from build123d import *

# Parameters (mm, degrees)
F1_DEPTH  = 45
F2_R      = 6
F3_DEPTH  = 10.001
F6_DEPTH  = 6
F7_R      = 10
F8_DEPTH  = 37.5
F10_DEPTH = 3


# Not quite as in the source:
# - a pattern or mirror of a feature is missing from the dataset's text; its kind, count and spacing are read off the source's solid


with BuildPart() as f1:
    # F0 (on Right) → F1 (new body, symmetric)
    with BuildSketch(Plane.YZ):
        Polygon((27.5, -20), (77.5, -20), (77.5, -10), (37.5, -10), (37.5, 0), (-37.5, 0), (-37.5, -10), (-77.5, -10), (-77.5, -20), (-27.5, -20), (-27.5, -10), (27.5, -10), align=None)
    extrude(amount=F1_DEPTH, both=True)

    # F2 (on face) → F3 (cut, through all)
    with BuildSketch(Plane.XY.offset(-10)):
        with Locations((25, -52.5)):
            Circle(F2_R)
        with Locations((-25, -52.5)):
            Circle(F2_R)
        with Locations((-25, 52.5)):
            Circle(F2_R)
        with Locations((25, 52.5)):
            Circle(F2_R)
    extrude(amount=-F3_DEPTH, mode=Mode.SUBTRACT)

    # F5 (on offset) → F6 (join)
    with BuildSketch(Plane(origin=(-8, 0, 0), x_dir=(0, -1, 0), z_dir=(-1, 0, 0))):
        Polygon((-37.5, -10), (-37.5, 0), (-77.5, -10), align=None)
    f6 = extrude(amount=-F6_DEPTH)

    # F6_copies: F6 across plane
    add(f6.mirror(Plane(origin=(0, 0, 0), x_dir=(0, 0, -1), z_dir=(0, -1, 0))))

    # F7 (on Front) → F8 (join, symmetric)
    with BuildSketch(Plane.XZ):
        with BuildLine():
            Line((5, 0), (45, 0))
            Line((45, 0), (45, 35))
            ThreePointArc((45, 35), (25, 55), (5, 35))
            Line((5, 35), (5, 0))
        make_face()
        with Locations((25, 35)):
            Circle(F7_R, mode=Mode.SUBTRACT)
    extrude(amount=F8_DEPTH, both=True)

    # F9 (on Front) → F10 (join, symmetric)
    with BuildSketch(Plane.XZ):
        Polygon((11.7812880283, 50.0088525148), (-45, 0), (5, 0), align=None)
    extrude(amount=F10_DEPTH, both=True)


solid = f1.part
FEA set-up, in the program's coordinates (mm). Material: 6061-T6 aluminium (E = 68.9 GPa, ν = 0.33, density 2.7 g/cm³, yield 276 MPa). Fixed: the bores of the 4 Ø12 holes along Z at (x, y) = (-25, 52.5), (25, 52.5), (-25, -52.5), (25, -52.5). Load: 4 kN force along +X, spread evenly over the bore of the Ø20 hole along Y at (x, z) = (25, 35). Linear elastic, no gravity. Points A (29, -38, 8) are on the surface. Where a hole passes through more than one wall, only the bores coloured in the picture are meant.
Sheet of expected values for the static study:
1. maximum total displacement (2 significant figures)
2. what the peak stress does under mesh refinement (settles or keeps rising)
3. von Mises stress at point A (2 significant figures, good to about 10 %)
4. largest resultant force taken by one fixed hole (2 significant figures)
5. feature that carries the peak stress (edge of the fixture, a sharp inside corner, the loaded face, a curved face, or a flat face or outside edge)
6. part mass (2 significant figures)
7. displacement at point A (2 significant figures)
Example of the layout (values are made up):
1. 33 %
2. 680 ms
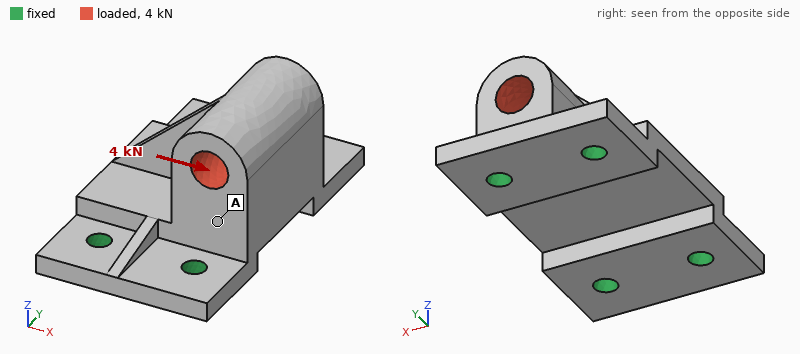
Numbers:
1. 54 µm
2. keeps rising
3. 4.0 MPa
4. 3.3 kN
5. edge of the fixture
6. 780 g
7. 20 µm
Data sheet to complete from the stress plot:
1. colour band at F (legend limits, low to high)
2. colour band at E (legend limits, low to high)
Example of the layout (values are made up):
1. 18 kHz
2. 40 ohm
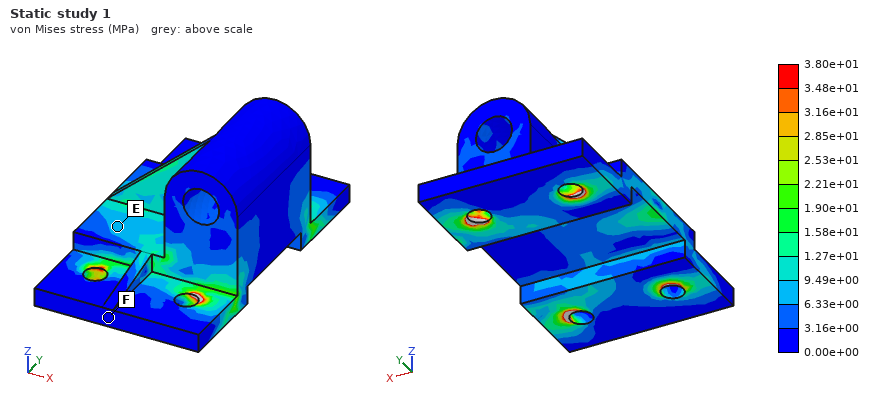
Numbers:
1. 0.00e+00 to 3.16e+00 MPa
2. 6.33e+00 to 9.49e+00 MPa
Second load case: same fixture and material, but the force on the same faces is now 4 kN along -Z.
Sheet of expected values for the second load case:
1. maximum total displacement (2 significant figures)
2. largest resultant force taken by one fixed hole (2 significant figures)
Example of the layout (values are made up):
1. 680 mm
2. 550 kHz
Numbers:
1. 16 µm
2. 2.3 kN
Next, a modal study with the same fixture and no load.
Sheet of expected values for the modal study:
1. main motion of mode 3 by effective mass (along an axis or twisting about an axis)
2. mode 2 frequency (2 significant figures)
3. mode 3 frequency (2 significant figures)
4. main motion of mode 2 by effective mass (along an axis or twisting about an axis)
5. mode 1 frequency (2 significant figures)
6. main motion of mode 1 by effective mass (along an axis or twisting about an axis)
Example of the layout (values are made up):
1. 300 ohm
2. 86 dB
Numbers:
1. along Z
2. 5000 Hz
3. 5200 Hz
4. along Y
5. 2900 Hz
6. along X
